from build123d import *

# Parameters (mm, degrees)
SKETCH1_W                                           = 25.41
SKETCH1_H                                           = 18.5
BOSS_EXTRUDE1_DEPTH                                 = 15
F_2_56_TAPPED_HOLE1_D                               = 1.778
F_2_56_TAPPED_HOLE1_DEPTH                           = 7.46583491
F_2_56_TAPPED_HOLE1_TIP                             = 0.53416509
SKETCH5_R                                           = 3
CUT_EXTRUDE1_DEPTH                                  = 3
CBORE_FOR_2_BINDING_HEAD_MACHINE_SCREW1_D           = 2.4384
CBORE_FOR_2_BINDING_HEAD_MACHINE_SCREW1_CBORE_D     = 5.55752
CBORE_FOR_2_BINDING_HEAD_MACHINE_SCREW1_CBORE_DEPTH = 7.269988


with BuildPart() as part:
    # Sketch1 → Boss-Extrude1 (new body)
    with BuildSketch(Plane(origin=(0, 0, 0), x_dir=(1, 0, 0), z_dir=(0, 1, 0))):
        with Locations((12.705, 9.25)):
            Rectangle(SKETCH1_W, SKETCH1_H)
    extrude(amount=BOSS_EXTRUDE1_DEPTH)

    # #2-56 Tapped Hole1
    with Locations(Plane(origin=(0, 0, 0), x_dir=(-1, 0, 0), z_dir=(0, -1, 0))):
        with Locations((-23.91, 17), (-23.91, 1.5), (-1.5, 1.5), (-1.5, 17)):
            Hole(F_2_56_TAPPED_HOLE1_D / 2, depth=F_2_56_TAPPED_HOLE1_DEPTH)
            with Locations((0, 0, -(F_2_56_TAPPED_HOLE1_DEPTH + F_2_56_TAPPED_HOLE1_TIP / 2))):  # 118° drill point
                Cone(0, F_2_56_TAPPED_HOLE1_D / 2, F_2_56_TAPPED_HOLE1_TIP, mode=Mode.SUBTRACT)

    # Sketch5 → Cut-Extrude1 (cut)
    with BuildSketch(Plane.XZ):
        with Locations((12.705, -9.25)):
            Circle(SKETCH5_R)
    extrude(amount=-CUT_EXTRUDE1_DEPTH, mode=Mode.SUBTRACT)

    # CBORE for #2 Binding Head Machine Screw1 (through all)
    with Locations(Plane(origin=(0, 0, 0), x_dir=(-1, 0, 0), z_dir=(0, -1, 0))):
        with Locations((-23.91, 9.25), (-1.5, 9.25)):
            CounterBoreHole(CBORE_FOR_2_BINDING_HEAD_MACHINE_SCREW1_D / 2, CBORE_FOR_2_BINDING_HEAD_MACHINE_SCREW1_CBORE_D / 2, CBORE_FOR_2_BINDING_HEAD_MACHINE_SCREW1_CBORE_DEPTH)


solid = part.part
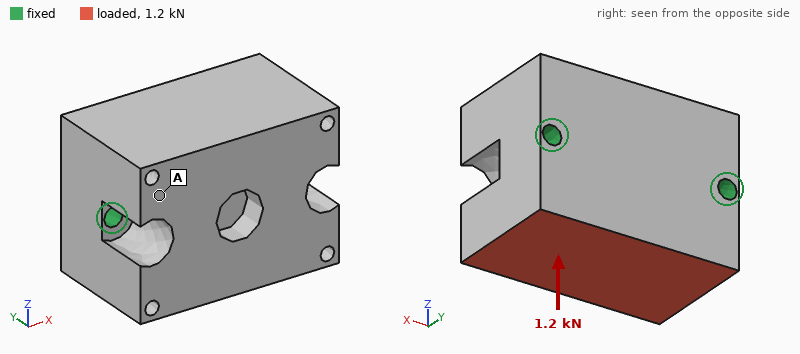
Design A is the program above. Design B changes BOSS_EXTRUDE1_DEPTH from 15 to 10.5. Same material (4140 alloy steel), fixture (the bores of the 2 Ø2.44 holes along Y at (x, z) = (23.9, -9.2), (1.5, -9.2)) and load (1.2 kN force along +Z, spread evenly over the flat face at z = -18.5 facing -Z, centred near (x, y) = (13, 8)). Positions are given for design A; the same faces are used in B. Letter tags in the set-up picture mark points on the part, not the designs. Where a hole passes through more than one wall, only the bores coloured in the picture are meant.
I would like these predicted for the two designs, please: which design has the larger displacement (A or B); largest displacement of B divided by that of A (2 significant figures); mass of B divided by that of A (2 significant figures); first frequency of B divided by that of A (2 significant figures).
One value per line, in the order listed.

B
4.6
0.68
0.52
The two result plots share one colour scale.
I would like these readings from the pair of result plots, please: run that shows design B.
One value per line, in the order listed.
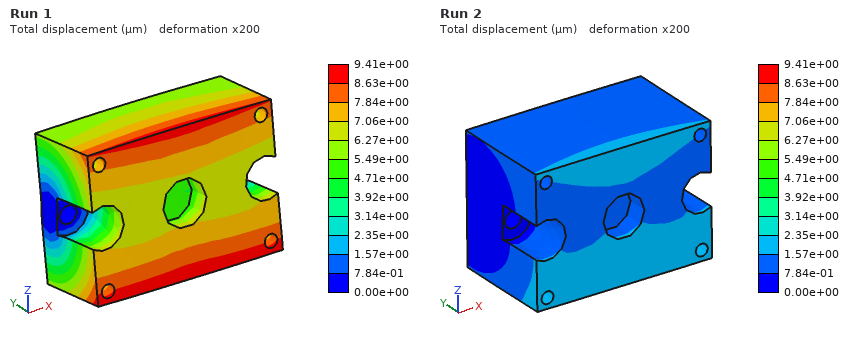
Run 1
